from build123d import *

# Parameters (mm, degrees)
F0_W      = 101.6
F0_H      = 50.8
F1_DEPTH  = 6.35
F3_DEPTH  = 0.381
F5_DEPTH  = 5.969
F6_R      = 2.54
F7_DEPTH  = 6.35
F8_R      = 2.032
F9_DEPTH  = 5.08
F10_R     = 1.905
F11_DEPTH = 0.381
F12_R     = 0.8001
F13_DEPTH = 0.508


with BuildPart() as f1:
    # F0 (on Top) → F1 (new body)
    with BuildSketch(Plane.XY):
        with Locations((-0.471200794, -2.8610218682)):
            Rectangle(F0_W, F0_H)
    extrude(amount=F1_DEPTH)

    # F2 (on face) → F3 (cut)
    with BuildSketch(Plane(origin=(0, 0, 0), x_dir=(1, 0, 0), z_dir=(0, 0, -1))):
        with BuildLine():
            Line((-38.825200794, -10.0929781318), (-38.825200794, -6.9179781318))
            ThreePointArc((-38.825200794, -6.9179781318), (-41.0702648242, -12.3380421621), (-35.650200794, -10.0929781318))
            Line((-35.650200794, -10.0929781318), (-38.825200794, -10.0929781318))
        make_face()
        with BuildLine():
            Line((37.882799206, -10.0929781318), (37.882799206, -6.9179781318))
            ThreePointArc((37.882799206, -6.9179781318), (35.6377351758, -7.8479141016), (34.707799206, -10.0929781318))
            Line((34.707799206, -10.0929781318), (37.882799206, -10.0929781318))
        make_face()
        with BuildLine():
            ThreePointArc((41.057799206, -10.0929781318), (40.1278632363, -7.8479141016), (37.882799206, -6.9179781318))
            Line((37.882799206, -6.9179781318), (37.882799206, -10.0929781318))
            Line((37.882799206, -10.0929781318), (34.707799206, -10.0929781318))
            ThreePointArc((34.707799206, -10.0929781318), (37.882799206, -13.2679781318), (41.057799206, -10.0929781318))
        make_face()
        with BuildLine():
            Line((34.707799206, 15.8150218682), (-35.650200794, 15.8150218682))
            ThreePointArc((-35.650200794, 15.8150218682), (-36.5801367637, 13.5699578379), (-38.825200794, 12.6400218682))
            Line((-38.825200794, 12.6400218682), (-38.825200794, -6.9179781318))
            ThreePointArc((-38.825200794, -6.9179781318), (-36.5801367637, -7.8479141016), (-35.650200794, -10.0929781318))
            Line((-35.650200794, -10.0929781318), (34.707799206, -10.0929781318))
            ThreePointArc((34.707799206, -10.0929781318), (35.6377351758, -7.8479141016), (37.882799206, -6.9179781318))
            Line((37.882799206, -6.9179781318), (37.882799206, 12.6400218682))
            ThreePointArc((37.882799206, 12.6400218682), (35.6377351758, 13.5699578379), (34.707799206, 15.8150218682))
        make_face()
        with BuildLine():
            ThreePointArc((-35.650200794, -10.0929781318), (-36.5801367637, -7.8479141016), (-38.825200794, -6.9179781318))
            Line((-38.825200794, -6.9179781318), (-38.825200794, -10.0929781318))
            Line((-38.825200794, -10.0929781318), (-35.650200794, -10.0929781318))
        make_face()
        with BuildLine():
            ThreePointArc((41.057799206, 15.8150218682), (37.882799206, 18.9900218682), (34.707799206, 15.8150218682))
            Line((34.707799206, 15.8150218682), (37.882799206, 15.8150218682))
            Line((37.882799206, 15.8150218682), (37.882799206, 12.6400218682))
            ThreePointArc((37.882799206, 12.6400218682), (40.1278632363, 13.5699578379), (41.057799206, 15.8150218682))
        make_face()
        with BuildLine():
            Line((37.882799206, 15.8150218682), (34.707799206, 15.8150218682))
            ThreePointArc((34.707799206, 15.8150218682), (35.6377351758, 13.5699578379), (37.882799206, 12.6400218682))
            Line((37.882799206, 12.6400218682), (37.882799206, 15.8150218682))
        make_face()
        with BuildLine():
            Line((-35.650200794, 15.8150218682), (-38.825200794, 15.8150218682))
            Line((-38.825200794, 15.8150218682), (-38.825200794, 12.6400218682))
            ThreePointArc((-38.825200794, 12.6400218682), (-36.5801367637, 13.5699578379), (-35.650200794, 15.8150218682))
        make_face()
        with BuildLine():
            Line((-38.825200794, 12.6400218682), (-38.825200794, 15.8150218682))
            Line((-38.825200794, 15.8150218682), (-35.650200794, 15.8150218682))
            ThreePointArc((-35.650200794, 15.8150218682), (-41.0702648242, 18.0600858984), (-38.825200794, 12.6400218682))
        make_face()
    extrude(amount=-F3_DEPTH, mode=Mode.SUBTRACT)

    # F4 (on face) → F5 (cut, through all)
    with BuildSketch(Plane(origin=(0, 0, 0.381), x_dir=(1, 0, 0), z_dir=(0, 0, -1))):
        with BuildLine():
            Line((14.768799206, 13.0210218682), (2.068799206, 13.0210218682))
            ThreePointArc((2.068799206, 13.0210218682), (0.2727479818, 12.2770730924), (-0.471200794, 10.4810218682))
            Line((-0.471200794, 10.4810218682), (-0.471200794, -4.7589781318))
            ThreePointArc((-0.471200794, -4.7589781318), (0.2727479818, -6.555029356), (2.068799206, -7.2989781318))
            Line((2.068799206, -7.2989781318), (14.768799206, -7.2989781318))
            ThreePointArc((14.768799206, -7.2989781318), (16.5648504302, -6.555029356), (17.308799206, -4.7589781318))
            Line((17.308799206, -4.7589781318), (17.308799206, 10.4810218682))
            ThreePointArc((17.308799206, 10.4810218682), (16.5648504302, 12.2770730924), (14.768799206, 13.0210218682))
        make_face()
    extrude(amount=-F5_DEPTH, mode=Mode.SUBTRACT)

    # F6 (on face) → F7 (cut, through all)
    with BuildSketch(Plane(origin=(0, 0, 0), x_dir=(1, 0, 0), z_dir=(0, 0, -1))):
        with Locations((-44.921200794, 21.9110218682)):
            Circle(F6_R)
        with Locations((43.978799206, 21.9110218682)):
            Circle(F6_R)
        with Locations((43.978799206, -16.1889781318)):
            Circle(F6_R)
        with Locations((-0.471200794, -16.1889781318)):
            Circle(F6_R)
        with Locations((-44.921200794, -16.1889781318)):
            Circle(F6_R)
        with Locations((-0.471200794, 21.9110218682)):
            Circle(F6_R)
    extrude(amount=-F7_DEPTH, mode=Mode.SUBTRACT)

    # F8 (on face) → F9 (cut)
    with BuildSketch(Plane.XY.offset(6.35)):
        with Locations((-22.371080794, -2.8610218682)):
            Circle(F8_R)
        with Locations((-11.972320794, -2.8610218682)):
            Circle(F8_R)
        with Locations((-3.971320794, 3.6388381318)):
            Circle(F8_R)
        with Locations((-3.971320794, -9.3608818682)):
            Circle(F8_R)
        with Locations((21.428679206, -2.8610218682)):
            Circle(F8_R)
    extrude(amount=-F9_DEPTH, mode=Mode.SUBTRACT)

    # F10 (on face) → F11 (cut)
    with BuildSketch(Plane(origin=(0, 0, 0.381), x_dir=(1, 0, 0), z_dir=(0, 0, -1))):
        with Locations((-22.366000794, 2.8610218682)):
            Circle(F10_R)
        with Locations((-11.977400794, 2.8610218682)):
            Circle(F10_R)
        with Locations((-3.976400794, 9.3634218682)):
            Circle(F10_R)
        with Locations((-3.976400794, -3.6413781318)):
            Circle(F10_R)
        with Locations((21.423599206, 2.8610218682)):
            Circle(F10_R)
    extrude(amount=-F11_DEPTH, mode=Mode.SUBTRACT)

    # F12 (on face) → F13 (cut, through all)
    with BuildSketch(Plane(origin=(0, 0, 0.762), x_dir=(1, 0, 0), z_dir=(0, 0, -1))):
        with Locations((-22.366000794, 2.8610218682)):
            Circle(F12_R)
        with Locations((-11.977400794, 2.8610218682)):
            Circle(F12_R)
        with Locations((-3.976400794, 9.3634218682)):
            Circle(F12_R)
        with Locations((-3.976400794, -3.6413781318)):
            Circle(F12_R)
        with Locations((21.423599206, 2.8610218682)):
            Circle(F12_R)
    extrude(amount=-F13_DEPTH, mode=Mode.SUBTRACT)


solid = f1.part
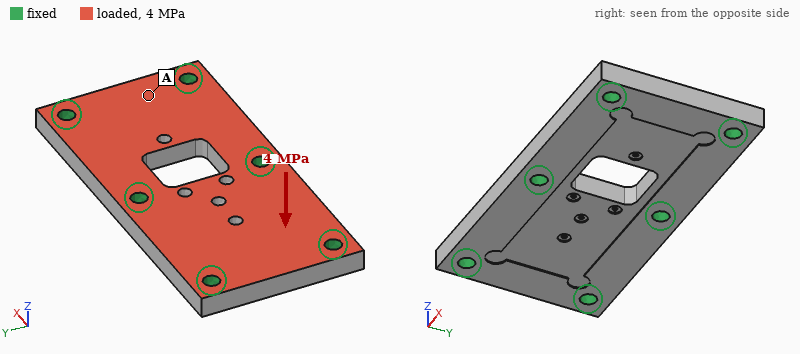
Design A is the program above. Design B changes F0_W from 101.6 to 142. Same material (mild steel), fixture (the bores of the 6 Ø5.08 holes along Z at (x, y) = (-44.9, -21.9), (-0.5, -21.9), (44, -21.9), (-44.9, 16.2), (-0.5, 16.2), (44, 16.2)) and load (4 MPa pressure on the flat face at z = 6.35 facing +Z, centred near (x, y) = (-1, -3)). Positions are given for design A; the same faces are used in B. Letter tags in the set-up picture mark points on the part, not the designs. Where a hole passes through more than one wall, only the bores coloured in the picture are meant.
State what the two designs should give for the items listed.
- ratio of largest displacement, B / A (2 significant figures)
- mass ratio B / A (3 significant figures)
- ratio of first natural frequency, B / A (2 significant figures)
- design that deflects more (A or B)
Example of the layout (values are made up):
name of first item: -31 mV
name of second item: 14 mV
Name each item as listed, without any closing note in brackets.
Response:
ratio of largest displacement, B / A: 3.2
mass ratio B / A: 1.45
ratio of first natural frequency, B / A: 0.53
design that deflects more: B
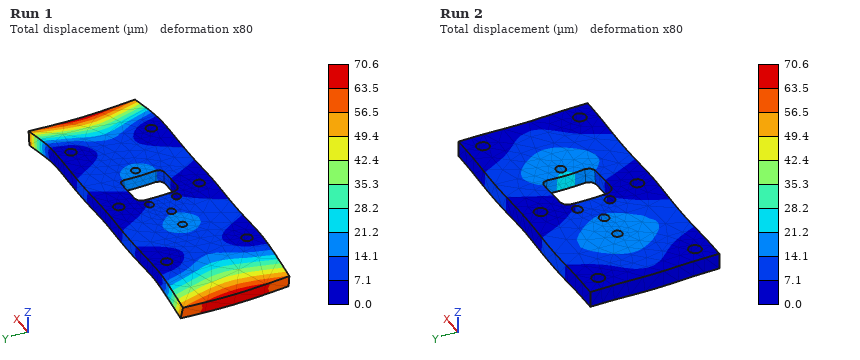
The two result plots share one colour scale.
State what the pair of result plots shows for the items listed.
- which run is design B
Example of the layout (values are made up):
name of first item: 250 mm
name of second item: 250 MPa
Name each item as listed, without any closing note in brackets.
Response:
which run is design B: Run 1
